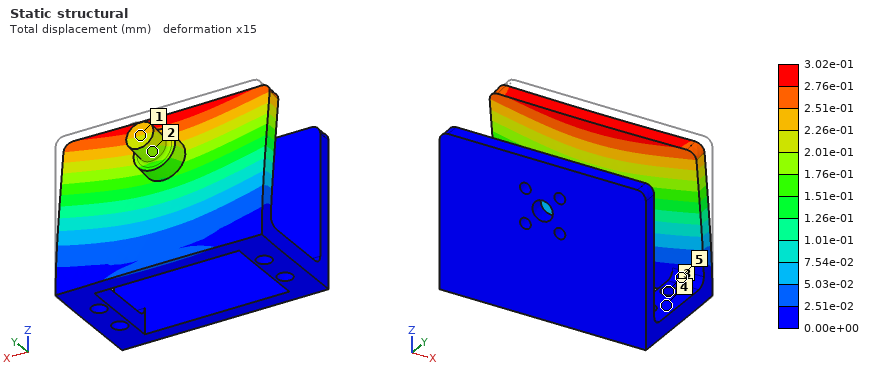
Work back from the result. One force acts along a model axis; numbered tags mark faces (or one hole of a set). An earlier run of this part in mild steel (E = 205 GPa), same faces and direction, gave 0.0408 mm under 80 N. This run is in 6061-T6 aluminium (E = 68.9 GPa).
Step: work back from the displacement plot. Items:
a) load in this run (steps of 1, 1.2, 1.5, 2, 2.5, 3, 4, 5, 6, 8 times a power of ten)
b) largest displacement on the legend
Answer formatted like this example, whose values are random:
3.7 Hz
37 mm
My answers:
200 N
3.02e-01 mm
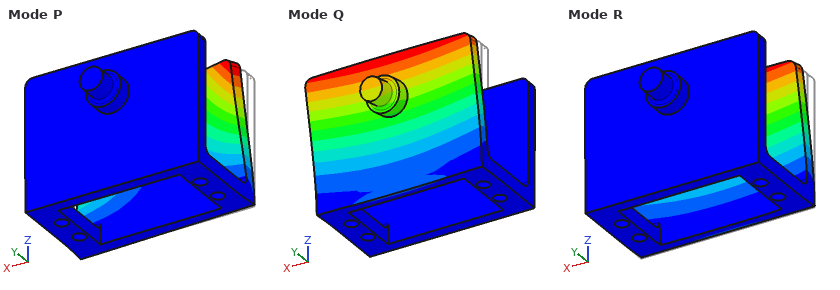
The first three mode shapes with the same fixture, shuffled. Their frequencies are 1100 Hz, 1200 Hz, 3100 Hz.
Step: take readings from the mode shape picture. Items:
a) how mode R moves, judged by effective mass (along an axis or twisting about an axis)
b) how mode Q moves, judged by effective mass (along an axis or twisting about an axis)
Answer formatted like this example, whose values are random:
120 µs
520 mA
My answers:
along Y
along Y
